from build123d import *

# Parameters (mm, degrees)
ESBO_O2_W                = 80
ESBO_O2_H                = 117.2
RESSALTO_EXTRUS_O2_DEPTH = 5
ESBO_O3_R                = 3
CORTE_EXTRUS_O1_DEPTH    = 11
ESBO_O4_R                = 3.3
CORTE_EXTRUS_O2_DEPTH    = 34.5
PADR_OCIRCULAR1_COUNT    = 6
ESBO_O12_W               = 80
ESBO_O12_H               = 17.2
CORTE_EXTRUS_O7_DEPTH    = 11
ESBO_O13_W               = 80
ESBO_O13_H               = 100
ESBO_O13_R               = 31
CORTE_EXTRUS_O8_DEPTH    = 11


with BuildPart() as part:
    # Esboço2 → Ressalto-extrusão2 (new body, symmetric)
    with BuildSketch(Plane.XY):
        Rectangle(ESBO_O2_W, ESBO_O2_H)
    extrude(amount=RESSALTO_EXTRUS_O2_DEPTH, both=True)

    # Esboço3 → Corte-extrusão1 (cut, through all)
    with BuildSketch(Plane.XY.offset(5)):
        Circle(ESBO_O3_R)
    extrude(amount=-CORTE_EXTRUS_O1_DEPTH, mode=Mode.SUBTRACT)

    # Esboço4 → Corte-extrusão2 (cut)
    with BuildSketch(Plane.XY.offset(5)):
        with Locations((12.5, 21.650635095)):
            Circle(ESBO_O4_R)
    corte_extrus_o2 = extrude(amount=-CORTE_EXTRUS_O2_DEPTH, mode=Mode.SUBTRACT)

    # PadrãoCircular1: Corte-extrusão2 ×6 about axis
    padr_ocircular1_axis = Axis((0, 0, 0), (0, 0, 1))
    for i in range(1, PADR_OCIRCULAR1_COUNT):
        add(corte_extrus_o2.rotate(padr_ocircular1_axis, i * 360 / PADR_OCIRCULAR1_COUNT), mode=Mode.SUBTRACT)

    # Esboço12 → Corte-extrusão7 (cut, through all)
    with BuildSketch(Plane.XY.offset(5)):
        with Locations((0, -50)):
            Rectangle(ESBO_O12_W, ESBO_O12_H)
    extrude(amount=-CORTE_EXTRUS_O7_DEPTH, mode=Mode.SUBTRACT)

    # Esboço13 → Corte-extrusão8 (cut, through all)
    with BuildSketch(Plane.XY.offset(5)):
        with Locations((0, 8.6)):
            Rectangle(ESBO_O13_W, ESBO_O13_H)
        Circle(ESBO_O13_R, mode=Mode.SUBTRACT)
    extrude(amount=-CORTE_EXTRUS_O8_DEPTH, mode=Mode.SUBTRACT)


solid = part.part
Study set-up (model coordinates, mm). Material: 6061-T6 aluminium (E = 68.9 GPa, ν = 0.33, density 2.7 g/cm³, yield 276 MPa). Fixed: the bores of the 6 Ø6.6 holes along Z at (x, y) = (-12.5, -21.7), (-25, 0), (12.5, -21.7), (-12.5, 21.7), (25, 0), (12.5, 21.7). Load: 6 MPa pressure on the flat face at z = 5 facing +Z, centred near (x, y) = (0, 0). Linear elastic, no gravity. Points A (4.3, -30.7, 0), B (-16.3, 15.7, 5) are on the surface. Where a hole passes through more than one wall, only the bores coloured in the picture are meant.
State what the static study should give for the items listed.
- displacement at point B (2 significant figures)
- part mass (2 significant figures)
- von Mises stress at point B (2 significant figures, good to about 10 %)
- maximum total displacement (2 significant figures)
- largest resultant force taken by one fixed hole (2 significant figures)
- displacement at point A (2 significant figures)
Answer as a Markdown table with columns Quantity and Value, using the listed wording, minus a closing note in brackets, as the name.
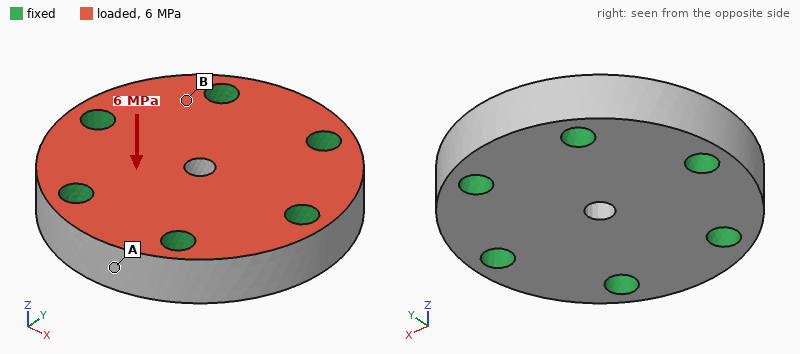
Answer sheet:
| Quantity | Value |
|---|---|
| displacement at point B | 2.5 µm |
| part mass | 75 g |
| von Mises stress at point B | 13 MPa |
| maximum total displacement | 10 µm |
| largest resultant force taken by one fixed hole | 2.8 kN |
| displacement at point A | 2.0 µm |
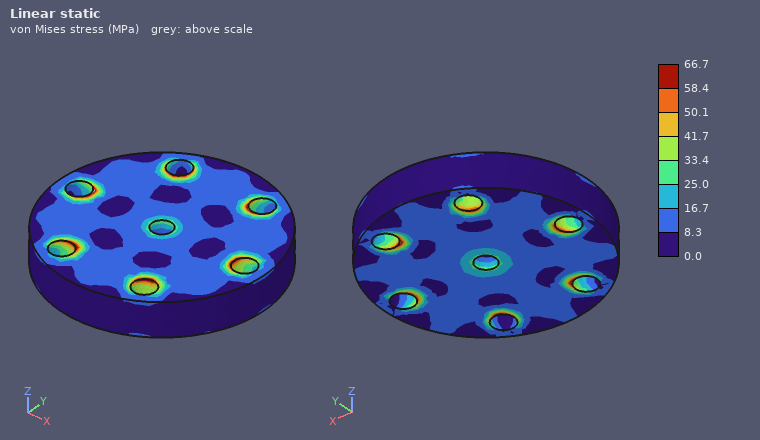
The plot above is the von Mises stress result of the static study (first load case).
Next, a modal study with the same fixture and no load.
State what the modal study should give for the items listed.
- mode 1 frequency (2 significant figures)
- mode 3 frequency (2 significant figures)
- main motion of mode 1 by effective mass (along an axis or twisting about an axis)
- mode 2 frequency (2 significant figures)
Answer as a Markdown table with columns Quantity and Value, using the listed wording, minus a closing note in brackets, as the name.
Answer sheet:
| Quantity | Value |
|---|---|
| mode 1 frequency | 29 kHz |
| mode 3 frequency | 48 kHz |
| main motion of mode 1 by effective mass | along Z |
| mode 2 frequency | 48 kHz |
